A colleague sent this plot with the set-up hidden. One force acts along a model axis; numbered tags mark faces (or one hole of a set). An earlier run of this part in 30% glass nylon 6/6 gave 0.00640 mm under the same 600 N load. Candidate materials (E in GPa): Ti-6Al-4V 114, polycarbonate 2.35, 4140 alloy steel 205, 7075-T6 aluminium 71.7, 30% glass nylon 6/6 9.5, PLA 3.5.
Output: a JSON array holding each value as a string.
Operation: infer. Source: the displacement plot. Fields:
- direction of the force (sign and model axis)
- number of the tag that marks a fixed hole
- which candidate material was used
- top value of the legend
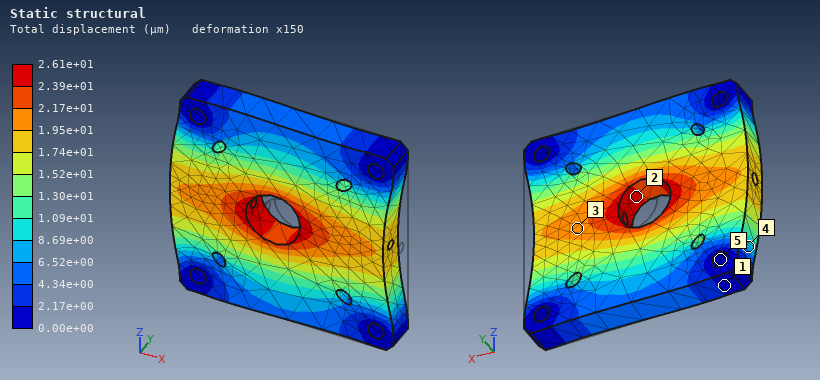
["-X", "5", "polycarbonate", "2.61e+01 µm"]
